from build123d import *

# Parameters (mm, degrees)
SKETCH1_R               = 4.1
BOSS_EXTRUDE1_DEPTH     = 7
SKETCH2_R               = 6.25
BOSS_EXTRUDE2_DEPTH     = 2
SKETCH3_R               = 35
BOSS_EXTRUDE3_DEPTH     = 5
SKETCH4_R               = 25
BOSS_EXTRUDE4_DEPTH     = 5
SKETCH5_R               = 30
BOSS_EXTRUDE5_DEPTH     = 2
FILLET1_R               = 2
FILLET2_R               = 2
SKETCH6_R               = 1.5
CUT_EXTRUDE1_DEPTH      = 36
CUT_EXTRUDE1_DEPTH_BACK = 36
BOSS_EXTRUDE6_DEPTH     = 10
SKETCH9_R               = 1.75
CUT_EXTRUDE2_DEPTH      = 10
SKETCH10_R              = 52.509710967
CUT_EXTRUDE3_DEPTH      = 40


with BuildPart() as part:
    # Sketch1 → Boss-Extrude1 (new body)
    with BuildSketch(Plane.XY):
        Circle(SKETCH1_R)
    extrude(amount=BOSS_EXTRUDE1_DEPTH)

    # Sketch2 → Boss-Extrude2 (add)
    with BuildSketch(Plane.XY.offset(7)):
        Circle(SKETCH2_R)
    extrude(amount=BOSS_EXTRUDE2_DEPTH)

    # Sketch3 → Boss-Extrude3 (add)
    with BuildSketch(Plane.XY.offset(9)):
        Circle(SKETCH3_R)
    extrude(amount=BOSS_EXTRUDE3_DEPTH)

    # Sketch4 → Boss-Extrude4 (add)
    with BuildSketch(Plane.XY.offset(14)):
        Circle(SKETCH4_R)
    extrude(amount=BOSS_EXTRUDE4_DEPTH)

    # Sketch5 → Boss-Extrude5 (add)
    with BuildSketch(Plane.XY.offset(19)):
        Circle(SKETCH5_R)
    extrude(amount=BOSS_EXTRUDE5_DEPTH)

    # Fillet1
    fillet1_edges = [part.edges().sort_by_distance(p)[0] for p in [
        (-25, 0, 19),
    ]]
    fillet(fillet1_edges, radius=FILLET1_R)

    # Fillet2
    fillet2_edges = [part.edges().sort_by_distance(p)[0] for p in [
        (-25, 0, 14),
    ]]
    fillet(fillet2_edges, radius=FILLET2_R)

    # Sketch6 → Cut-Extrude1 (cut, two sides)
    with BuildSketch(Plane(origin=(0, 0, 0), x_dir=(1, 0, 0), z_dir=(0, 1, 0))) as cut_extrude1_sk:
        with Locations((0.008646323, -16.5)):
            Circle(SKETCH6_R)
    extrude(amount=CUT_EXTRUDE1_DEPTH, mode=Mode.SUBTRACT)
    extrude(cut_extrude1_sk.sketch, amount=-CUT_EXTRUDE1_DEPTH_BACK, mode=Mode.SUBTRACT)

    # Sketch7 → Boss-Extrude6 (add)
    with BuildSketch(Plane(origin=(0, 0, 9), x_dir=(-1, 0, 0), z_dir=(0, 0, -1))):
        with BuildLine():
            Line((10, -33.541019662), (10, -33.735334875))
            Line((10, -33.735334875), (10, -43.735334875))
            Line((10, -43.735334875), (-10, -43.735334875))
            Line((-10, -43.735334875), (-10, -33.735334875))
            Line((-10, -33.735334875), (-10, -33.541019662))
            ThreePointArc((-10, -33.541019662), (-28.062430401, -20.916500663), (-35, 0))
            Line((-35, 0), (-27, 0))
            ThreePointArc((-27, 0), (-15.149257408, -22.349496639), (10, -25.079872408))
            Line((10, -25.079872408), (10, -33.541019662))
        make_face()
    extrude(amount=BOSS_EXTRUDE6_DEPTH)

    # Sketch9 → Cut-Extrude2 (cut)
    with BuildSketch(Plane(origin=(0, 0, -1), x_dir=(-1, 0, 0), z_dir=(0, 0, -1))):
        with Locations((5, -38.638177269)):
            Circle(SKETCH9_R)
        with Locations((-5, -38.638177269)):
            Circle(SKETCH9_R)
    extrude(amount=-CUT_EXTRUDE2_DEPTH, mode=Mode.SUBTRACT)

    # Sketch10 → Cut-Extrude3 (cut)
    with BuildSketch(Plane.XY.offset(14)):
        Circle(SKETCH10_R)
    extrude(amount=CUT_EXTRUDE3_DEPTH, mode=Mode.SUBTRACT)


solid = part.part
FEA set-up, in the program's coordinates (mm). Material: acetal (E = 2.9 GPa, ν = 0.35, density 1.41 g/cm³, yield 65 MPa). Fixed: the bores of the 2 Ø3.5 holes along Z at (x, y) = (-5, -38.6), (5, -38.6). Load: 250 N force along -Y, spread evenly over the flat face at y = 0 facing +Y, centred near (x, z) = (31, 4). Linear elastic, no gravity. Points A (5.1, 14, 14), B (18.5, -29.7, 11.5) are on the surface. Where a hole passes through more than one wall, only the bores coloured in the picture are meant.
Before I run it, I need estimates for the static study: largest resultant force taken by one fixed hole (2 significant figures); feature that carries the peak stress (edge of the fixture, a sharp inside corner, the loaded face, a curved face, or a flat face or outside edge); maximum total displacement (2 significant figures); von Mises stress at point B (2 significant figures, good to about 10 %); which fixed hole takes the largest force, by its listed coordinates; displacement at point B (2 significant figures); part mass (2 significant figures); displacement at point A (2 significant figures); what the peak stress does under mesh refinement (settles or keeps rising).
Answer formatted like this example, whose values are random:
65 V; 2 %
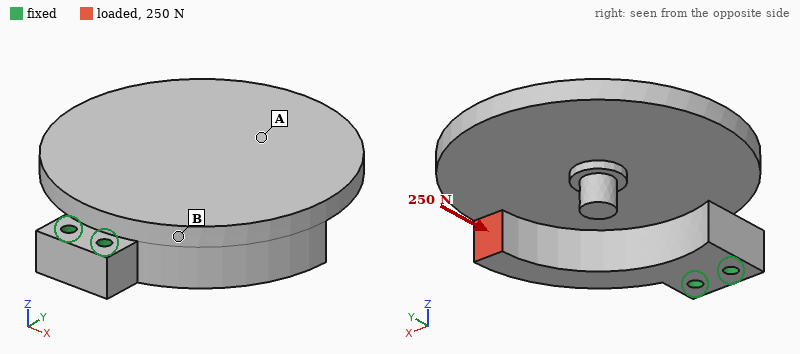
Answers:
770 N; edge of the fixture; 0.69 mm; 4.3 MPa; (5, -38.6); 0.17 mm; 37 g; 0.45 mm; keeps rising
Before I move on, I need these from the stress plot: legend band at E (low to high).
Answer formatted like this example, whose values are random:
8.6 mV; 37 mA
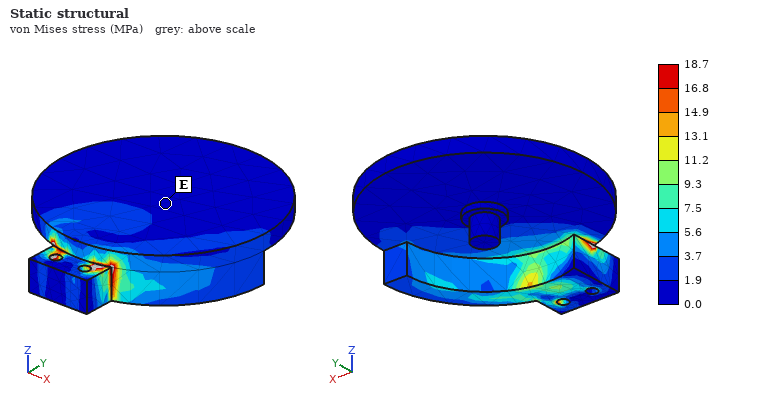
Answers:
0.0 to 1.9 MPa
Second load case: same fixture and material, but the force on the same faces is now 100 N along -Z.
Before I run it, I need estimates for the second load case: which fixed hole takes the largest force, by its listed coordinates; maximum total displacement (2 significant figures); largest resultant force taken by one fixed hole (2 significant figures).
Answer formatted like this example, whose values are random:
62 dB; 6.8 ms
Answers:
(5, -38.6); 1.1 mm; 190 N
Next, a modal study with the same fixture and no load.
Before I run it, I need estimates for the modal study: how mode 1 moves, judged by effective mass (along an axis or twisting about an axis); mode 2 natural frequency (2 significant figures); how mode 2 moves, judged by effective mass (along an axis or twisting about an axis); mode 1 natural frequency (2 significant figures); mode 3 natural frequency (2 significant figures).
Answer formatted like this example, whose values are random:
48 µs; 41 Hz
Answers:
along Z; 570 Hz; along X; 300 Hz; 750 Hz
